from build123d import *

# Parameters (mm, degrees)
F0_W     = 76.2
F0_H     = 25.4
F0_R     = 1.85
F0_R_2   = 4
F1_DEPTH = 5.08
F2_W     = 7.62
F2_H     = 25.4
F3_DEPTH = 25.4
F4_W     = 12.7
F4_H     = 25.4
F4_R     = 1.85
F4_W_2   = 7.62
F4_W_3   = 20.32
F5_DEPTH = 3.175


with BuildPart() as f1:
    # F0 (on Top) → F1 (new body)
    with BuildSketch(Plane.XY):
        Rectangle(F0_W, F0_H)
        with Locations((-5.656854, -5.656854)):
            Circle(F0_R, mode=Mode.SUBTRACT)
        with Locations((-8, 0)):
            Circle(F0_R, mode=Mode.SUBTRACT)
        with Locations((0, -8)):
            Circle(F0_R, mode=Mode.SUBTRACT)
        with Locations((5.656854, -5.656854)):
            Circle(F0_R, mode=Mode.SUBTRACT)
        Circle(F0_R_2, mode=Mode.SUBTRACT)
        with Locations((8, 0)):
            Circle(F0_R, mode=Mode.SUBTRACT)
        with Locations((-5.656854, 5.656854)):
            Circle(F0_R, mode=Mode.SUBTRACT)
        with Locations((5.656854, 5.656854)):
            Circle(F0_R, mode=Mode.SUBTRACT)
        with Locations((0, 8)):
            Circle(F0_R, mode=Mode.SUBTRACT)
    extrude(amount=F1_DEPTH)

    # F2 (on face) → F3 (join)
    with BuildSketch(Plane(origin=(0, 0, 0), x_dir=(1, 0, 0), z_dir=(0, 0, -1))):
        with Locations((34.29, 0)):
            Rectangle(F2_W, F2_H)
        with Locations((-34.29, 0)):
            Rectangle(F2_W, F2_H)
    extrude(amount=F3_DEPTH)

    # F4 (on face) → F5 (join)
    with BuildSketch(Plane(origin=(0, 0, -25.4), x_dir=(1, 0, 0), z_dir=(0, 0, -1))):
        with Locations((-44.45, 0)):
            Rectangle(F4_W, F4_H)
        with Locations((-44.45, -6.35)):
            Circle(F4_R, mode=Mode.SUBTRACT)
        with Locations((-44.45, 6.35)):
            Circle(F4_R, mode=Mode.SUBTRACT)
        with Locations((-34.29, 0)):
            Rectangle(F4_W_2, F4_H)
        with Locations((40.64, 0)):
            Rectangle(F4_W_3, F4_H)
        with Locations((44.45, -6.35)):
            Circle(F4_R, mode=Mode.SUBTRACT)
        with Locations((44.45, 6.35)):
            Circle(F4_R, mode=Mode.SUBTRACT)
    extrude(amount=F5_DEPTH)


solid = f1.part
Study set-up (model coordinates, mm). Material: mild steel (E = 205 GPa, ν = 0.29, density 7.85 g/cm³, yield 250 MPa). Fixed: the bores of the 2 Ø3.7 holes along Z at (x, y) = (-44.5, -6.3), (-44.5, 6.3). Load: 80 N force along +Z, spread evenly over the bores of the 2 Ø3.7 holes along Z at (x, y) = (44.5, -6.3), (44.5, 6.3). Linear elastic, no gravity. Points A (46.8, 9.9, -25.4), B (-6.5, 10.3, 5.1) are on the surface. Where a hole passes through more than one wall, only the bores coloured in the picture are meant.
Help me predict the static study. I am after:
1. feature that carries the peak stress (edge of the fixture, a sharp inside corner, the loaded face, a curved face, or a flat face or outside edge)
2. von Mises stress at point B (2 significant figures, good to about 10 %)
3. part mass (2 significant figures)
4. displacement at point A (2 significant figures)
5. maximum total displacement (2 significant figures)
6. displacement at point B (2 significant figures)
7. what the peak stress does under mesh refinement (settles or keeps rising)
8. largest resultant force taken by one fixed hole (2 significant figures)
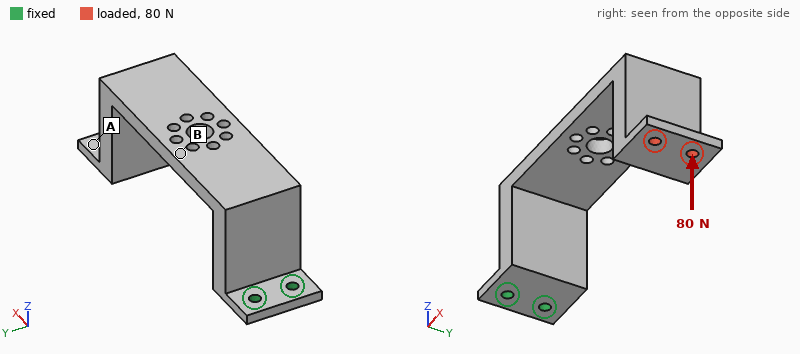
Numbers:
edge of the fixture
57 MPa
170 g
0.66 mm
0.70 mm
0.22 mm
keeps rising
51 N
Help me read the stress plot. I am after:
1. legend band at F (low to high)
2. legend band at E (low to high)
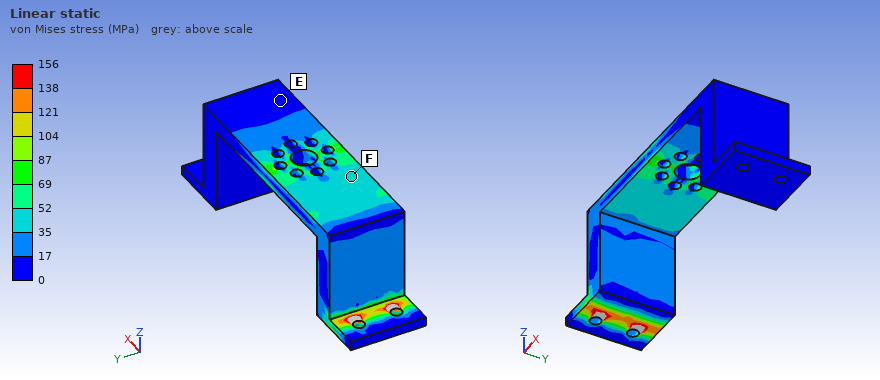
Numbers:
35 to 52 MPa
0 to 17 MPa
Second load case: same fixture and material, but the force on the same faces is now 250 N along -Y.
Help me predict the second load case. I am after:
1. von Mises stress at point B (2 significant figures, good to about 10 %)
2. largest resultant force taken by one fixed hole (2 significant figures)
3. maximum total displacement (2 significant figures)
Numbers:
90 MPa
1.5 kN
0.51 mm
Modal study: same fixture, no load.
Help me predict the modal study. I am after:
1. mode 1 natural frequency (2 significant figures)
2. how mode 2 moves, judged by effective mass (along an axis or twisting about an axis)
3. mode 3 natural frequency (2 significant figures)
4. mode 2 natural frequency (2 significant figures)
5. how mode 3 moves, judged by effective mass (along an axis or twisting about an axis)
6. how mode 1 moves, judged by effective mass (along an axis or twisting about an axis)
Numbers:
230 Hz
along Y
750 Hz
600 Hz
along X
along Z
